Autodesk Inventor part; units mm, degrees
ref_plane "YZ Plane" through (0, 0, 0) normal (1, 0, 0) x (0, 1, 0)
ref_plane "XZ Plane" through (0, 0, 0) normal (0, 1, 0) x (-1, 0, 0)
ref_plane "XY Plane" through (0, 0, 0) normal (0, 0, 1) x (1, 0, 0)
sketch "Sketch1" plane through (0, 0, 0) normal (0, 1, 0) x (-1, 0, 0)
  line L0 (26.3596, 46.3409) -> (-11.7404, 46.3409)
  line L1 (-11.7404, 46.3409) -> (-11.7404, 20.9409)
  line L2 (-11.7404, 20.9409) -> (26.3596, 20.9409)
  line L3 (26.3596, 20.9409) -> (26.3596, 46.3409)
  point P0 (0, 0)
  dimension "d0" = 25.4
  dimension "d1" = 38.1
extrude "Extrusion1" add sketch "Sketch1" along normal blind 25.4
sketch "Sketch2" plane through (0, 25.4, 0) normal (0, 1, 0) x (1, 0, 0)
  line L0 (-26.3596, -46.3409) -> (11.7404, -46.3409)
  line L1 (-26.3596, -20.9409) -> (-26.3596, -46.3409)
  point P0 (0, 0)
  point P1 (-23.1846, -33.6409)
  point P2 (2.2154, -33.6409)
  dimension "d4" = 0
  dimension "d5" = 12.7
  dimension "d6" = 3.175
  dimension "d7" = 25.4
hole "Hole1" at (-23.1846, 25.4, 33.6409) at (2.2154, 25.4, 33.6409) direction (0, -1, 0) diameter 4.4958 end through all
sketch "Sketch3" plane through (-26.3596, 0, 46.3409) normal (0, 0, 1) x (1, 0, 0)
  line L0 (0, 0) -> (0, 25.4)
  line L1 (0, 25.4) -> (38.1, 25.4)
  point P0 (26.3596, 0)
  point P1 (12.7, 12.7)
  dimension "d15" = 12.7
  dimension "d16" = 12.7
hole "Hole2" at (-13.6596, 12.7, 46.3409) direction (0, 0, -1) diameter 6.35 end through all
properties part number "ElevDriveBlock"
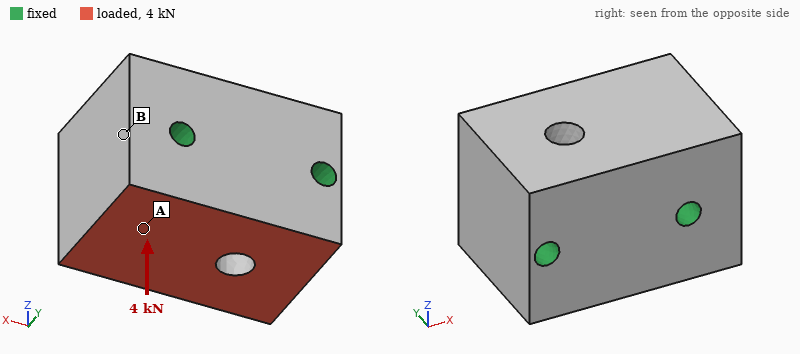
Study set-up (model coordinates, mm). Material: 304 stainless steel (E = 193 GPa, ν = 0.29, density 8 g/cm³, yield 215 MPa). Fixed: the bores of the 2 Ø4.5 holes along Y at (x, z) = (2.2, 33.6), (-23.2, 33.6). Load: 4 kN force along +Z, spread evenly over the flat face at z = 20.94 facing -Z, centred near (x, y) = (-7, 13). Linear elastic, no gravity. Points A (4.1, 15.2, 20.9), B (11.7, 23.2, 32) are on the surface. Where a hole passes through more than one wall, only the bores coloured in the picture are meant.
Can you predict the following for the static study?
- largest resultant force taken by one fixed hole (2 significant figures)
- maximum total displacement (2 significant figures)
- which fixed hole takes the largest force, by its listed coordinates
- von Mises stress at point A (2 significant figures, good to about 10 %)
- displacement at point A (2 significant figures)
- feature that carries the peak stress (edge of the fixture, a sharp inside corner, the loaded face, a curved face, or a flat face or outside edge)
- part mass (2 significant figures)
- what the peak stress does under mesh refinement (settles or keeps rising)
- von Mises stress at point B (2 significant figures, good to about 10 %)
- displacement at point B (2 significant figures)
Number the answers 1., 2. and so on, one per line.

1. 2.5 kN
2. 0.48 µm
3. (2.2, 33.6)
4. 5.5 MPa
5. 0.35 µm
6. edge of the fixture
7. 180 g
8. keeps rising
9. 2.5 MPa
10. 0.25 µm
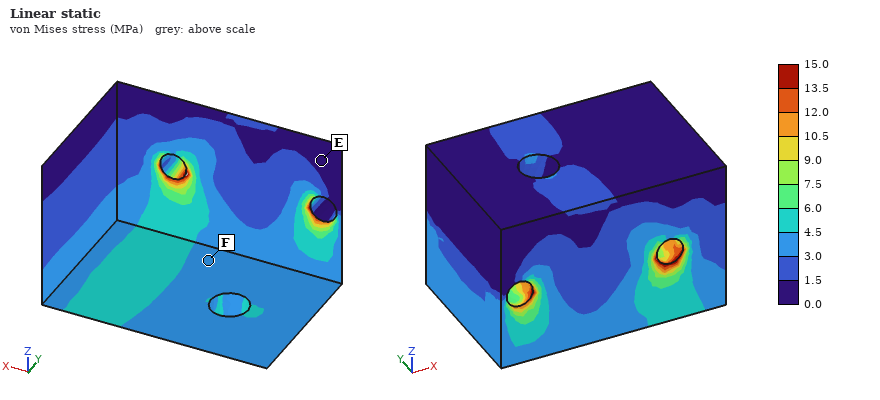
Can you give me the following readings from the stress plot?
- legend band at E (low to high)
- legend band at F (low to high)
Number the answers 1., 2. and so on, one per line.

1. 0.0 to 1.5 MPa
2. 3.0 to 4.5 MPa
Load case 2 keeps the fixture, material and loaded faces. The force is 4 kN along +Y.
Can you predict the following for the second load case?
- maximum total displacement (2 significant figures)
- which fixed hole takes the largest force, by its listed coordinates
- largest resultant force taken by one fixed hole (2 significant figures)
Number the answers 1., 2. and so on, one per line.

1. 2.0 µm
2. (2.2, 33.6)
3. 2.4 kN
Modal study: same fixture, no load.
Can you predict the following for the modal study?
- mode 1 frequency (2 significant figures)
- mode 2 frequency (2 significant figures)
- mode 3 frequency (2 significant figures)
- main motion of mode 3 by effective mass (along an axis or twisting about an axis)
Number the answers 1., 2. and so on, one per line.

1. 40 kHz
2. 40 kHz
3. 42 kHz
4. along Y
